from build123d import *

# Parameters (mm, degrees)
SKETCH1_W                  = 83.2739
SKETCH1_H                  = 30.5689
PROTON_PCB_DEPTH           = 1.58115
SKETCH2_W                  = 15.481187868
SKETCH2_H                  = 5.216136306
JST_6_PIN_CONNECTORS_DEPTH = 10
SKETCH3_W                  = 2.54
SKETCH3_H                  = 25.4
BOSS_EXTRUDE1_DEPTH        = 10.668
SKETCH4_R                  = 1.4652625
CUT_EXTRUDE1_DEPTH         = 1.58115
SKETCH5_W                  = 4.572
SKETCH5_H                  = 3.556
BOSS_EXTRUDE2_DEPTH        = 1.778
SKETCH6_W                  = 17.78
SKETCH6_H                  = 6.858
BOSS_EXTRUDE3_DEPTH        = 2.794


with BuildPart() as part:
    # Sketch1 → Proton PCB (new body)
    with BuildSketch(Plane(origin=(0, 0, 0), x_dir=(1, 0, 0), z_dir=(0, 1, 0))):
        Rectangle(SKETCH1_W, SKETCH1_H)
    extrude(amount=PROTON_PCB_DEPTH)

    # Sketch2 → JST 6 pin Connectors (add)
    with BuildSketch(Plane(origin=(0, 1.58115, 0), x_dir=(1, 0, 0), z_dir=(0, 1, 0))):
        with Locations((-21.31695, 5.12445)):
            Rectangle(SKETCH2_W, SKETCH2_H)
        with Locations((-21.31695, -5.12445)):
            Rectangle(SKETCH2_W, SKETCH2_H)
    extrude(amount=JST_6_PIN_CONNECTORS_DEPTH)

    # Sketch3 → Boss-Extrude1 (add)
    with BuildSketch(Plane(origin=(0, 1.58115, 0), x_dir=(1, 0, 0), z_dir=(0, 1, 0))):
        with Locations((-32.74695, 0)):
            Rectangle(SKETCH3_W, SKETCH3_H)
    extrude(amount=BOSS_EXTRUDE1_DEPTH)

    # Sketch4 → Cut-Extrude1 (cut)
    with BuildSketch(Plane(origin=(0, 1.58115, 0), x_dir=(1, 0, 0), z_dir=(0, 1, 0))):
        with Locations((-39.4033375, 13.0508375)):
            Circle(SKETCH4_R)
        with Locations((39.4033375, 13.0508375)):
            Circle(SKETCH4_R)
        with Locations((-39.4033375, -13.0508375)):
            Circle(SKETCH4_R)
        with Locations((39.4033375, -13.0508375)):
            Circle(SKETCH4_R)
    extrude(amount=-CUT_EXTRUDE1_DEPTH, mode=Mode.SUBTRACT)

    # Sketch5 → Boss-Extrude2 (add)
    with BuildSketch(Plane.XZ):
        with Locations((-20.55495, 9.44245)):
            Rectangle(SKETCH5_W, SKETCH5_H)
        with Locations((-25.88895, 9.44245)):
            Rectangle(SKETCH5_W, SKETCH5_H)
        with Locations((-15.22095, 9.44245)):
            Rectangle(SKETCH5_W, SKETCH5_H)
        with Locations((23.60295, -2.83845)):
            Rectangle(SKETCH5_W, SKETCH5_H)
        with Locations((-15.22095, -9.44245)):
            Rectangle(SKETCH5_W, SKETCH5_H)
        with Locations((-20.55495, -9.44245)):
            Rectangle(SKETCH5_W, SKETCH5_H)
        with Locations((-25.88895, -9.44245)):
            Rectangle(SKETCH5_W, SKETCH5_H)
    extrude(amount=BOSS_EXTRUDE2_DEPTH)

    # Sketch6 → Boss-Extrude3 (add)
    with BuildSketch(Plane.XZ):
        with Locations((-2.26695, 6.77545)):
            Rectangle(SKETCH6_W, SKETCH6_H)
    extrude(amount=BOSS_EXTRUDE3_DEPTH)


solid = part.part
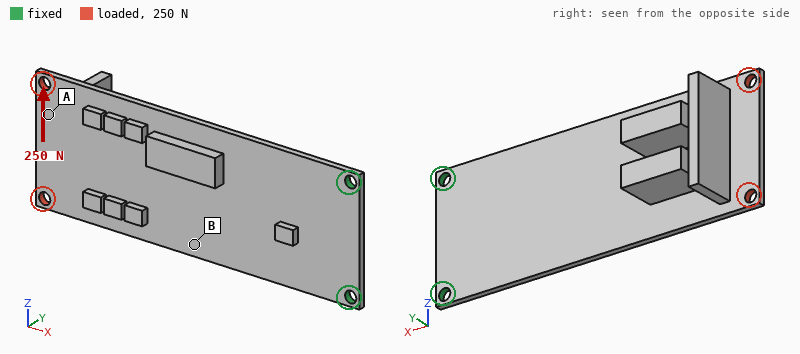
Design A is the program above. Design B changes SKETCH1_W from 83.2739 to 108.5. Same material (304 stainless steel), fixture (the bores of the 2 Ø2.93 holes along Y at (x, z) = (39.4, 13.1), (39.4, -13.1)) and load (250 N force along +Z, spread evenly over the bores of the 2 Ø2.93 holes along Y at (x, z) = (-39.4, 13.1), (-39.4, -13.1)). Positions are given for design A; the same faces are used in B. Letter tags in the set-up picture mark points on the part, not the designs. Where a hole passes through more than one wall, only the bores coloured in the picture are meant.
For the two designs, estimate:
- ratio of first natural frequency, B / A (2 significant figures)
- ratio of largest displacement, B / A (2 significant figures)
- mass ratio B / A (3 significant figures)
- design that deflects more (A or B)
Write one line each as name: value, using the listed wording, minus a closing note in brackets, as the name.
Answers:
ratio of first natural frequency, B / A: 0.90
ratio of largest displacement, B / A: 1.2
mass ratio B / A: 1.18
design that deflects more: B
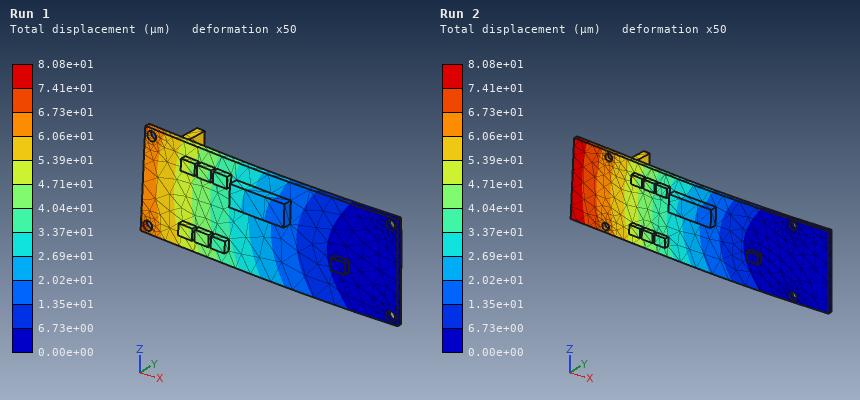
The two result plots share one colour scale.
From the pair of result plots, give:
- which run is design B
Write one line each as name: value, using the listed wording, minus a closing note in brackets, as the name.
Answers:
which run is design B: Run 2
